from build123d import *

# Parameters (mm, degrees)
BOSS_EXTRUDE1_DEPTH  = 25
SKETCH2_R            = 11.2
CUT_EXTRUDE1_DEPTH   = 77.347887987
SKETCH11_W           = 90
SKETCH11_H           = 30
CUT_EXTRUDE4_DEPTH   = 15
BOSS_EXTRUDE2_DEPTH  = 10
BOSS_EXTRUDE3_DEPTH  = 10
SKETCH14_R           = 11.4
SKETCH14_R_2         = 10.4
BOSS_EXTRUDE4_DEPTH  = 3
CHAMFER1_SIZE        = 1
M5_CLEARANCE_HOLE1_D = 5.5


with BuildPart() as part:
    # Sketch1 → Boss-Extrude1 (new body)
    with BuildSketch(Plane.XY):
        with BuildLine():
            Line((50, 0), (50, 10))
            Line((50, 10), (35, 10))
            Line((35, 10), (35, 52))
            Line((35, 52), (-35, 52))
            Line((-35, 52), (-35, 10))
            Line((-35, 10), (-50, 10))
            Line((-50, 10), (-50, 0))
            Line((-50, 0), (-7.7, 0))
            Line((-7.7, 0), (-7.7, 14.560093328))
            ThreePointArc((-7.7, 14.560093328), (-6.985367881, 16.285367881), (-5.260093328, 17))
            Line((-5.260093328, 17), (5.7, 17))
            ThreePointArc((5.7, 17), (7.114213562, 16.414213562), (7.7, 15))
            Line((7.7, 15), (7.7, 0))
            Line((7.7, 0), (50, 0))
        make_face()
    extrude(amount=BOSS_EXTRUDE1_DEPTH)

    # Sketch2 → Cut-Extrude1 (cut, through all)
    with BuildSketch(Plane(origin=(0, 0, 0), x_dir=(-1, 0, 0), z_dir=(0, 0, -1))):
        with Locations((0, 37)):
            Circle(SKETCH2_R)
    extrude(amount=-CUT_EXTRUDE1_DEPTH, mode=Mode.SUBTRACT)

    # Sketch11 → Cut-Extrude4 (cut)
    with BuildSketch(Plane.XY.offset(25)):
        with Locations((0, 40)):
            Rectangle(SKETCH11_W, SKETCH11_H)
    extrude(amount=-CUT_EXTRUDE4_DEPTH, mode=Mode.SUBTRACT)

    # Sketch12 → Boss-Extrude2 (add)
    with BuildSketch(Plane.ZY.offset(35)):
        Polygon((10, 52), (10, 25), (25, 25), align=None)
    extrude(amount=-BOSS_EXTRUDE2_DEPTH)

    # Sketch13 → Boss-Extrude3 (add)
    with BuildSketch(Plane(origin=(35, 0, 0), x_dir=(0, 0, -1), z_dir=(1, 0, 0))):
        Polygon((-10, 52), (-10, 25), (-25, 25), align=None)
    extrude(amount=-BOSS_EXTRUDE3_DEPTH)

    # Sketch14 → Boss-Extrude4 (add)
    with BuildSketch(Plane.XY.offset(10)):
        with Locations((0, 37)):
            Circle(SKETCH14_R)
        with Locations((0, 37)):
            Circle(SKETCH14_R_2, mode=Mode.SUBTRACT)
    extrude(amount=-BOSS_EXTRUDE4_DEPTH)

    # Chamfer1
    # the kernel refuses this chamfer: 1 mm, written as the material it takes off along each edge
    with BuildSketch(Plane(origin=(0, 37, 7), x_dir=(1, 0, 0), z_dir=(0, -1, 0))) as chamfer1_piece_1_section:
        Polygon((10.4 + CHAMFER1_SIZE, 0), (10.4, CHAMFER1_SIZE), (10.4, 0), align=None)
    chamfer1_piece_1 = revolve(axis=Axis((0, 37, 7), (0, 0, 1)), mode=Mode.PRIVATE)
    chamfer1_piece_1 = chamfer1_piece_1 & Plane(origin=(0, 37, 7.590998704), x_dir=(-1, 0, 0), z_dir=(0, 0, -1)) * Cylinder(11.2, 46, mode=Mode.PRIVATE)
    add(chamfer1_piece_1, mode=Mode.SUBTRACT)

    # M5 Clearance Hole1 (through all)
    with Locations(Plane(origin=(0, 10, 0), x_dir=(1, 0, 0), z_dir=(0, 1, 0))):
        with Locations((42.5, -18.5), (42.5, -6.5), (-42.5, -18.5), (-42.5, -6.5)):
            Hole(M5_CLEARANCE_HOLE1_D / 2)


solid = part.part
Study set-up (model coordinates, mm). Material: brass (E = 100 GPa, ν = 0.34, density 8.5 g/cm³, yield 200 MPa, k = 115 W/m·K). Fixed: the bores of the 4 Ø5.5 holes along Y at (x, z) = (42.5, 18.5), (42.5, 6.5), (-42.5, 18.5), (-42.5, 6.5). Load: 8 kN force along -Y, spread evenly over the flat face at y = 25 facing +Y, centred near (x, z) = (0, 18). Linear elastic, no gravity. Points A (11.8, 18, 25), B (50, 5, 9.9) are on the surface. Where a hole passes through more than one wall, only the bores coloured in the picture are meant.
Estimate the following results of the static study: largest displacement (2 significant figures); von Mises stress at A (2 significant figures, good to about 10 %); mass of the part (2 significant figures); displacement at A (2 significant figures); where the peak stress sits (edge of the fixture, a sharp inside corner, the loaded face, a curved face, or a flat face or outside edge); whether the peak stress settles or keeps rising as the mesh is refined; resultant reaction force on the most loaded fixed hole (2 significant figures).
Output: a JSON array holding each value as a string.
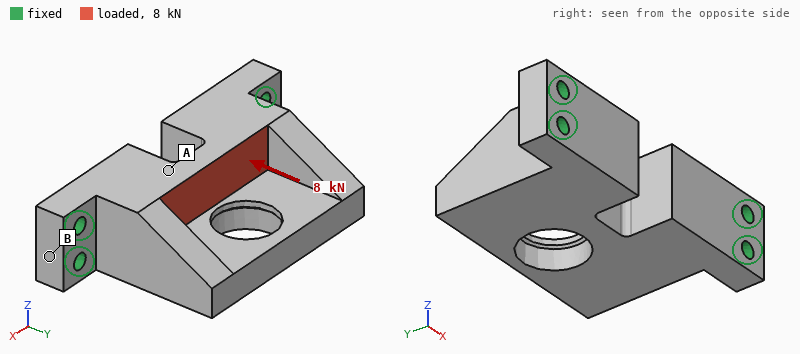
["30 µm", "20 MPa", "540 g", "24 µm", "edge of the fixture", "keeps rising", "3.6 kN"]
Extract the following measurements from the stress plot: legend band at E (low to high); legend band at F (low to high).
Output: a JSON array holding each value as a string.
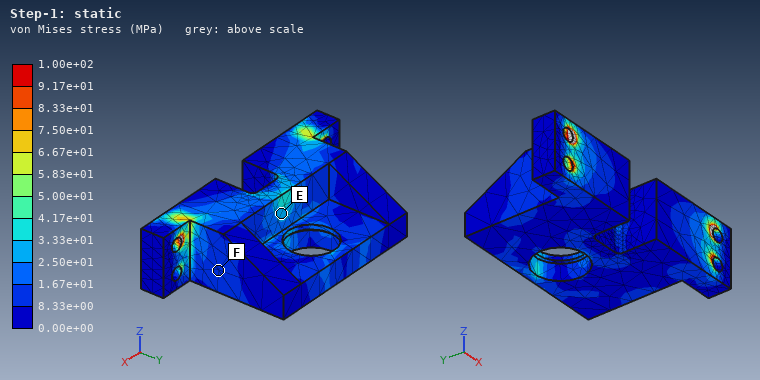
["2.50e+01 to 3.33e+01 MPa", "8.33e+00 to 1.67e+01 MPa"]
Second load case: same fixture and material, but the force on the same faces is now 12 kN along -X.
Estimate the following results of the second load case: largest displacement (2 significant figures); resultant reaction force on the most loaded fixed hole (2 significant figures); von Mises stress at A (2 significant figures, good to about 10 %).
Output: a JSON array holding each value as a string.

["19 µm", "3.5 kN", "25 MPa"]
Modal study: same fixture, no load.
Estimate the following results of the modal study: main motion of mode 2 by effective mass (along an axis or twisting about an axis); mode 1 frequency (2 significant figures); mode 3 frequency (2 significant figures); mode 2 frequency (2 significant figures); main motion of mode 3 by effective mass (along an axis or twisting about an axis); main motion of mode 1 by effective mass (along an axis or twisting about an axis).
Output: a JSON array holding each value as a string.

["twisting about Y", "2600 Hz", "6400 Hz", "4600 Hz", "along Y", "along Z"]
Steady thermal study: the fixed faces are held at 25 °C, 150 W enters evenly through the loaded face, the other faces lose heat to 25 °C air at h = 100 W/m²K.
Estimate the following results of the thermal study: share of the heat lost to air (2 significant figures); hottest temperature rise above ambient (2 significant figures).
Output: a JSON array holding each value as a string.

["25 %", "59 K"]
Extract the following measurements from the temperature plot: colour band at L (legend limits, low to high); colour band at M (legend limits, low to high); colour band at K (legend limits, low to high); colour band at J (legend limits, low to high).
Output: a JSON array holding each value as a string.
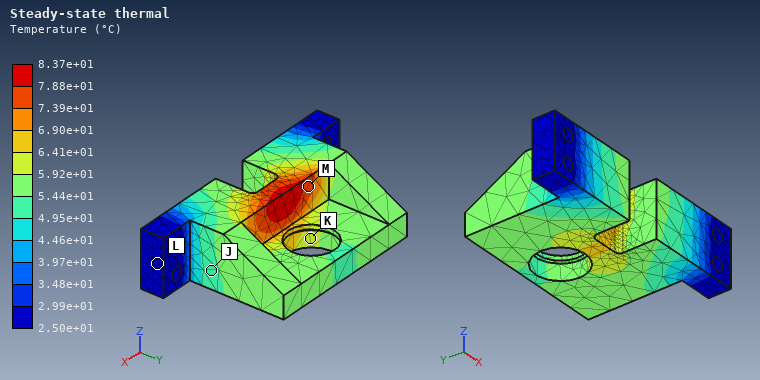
["2.50e+01 to 2.99e+01 °C", "7.39e+01 to 7.88e+01 °C", "5.92e+01 to 6.41e+01 °C", "4.95e+01 to 5.44e+01 °C"]
